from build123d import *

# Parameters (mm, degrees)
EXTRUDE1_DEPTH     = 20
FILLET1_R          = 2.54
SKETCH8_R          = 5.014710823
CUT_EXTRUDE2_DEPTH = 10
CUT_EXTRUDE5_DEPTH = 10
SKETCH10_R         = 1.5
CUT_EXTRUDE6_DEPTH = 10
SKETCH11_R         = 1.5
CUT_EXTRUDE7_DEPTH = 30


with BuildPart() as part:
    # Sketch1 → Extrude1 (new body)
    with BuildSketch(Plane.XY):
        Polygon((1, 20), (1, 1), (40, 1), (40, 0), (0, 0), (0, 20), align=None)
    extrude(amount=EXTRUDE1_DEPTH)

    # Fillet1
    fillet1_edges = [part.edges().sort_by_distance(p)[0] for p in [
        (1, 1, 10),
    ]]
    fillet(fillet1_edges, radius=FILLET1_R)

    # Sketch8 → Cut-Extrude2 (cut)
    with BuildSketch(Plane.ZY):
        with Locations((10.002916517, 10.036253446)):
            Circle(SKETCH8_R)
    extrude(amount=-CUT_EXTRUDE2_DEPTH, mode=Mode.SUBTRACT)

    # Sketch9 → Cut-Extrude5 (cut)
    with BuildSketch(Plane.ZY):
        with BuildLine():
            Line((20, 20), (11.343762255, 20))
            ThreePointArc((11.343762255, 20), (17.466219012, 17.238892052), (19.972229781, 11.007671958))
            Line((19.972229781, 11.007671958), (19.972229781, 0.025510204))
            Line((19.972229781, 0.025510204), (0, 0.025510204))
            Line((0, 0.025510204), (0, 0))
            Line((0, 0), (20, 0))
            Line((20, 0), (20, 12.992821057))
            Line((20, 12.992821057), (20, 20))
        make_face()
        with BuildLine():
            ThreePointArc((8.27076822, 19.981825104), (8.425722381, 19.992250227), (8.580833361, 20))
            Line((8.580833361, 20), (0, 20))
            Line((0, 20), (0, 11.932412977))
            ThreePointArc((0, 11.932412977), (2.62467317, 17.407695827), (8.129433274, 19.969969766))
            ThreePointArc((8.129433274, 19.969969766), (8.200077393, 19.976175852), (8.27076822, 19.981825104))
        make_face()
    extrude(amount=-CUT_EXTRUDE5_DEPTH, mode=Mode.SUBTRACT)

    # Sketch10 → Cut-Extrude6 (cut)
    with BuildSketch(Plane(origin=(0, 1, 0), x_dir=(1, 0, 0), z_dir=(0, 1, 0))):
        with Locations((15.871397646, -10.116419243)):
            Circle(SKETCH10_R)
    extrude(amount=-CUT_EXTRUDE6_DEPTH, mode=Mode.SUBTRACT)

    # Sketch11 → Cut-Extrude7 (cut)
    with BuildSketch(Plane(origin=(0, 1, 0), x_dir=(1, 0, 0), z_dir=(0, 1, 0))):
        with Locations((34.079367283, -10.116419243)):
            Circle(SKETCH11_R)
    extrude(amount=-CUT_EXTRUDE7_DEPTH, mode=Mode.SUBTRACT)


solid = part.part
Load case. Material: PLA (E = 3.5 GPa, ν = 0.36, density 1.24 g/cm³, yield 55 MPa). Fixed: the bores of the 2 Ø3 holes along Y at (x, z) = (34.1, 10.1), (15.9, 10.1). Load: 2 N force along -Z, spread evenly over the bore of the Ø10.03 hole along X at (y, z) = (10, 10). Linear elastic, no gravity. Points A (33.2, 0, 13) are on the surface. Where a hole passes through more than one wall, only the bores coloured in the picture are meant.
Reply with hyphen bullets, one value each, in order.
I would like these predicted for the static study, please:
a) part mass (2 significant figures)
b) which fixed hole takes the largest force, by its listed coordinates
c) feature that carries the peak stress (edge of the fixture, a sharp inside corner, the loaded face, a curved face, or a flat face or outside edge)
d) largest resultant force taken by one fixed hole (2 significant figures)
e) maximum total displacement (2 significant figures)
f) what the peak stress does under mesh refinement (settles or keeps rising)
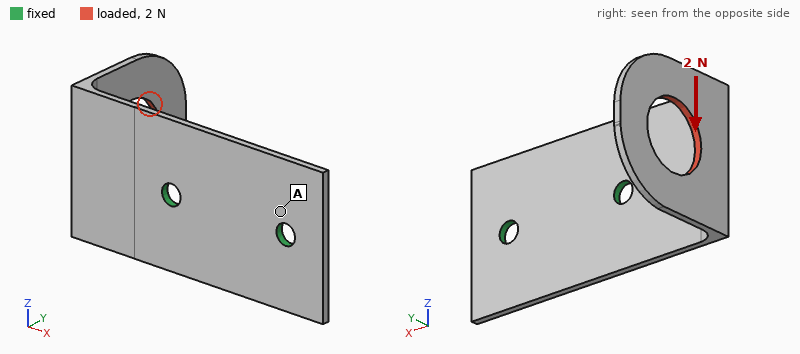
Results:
- 1.3 g
- (15.9, 10.1)
- edge of the fixture
- 3.3 N
- 0.48 mm
- keeps rising
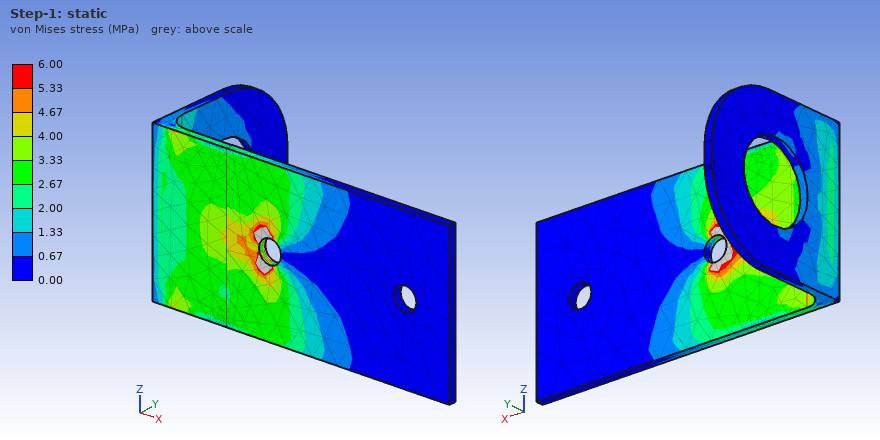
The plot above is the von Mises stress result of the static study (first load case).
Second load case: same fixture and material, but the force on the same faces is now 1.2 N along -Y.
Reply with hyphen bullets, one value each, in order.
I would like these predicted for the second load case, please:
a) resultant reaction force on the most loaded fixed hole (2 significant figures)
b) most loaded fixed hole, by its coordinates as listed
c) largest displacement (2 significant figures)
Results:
- 1.4 N
- (15.9, 10.1)
- 0.51 mm
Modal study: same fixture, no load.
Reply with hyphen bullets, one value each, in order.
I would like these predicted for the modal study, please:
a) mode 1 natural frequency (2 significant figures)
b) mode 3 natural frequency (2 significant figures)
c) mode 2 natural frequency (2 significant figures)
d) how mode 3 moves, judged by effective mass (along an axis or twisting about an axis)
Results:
- 370 Hz
- 990 Hz
- 590 Hz
- along Y
